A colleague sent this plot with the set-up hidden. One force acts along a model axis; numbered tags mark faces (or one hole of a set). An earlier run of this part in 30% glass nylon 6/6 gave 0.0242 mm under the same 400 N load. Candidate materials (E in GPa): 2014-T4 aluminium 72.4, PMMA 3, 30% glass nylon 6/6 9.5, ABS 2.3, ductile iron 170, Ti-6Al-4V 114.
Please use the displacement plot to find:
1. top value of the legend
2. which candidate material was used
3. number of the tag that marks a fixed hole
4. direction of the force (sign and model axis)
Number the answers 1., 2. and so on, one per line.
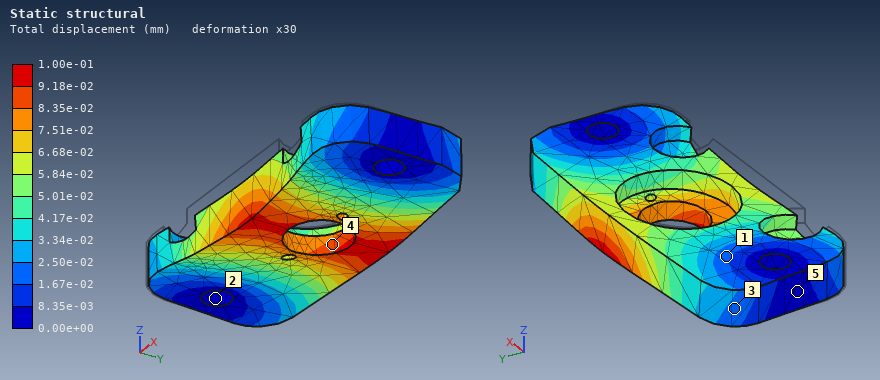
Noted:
1. 1.00e-01 mm
2. ABS
3. 2
4. +Y
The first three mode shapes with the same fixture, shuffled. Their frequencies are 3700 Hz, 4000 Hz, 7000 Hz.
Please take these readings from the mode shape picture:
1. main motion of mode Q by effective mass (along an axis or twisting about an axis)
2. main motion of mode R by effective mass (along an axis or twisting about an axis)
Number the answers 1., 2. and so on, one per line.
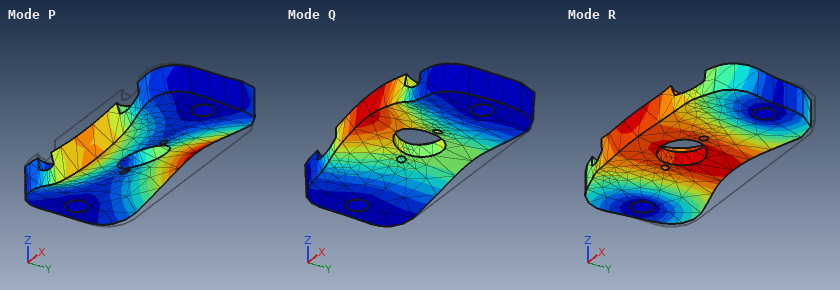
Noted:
1. along Z
2. along Y
